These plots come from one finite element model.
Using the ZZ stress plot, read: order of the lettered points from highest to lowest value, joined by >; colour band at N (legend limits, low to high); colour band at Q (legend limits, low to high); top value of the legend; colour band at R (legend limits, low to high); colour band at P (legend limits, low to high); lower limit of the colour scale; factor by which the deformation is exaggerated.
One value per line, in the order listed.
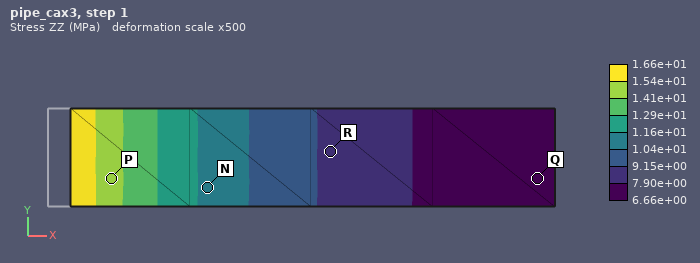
P > N > R > Q
1.04e+01 to 1.16e+01 MPa
6.66e+00 to 7.90e+00 MPa
1.66e+01 MPa
7.90e+00 to 9.15e+00 MPa
1.41e+01 to 1.54e+01 MPa
6.66e+00 MPa
500
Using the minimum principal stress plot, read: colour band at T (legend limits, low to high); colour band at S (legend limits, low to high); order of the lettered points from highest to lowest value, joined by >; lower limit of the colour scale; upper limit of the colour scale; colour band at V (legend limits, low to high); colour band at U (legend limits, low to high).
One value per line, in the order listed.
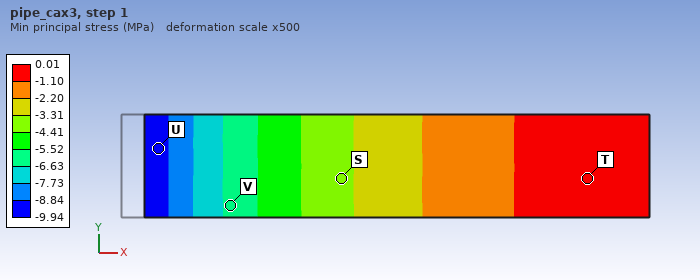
-1.10 to 0.01 MPa
-4.41 to -3.31 MPa
T > S > V > U
-9.94 MPa
0.01 MPa
-6.63 to -5.52 MPa
-9.94 to -8.84 MPa
